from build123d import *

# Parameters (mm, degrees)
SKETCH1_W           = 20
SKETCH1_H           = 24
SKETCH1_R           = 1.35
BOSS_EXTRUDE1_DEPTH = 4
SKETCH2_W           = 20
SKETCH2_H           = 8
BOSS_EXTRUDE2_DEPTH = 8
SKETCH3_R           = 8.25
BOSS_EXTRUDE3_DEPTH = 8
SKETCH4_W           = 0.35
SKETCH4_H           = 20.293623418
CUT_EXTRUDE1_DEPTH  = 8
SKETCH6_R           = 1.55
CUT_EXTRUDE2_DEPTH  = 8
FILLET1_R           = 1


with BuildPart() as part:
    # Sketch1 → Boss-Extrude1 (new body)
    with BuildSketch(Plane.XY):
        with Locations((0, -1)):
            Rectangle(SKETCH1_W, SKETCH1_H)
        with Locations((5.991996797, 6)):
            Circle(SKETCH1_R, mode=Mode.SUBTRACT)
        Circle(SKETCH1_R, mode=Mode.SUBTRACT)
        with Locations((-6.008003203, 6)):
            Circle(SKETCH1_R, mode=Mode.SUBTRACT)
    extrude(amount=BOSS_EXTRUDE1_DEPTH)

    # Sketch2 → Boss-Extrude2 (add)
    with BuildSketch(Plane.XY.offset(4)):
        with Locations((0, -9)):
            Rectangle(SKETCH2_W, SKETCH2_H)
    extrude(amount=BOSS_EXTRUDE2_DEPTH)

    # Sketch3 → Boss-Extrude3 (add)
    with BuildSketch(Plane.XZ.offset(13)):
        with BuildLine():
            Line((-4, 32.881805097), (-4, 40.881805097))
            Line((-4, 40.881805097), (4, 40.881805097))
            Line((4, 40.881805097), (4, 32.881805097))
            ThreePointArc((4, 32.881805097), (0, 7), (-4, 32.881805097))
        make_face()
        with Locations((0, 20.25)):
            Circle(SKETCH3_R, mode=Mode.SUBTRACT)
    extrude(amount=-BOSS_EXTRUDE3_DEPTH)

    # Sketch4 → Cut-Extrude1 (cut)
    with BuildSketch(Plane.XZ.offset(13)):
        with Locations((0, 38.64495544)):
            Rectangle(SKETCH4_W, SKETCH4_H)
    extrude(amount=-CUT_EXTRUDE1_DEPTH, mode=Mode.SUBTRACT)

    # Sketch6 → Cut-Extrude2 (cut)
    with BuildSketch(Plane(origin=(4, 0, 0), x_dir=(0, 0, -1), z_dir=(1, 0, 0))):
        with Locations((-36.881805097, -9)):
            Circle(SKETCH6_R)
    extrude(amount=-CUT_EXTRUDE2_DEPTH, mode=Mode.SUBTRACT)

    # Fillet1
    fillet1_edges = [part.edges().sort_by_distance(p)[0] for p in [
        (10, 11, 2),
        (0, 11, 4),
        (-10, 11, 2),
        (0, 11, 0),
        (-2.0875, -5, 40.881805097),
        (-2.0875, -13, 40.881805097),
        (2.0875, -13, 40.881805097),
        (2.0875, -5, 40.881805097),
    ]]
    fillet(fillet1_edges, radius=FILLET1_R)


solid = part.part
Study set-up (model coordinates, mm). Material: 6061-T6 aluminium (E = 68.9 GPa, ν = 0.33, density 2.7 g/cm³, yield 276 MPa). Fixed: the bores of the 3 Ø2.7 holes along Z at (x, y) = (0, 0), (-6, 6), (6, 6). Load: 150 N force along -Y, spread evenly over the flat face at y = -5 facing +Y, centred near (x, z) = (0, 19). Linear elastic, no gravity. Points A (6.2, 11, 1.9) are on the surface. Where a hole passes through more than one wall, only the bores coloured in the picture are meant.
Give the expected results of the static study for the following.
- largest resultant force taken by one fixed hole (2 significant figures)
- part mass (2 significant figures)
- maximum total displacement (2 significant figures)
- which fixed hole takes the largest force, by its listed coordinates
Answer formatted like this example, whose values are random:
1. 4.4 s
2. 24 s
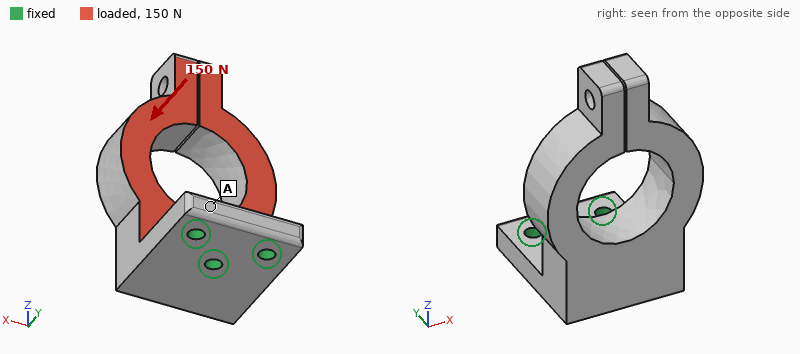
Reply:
1. 210 N
2. 15 g
3. 0.13 mm
4. (0, 0)
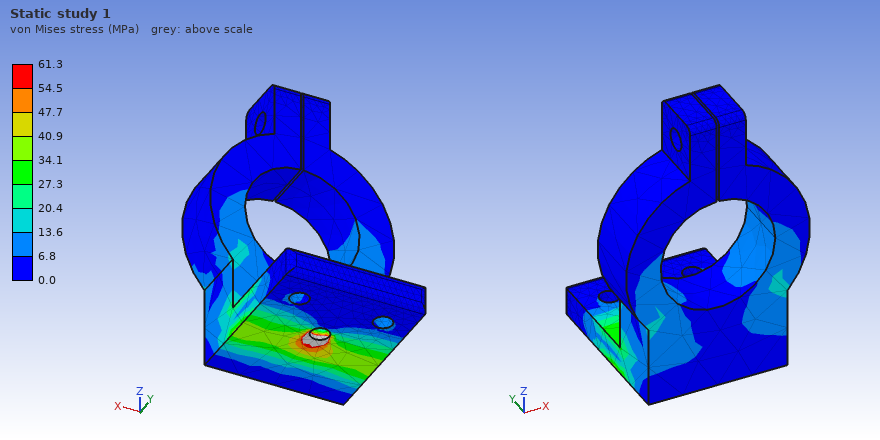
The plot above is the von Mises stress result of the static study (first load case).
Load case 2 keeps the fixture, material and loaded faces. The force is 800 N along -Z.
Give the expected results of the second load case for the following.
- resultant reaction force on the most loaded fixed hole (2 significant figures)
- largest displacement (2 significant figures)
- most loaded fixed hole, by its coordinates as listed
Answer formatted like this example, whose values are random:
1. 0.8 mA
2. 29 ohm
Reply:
1. 850 N
2. 62 µm
3. (0, 0)
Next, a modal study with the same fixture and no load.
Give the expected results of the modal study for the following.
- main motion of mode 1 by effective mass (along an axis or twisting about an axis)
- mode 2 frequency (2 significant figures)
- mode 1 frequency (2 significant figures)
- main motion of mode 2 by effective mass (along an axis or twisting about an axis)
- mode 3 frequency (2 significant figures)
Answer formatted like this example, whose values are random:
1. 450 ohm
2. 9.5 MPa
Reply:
1. along Y
2. 2700 Hz
3. 2100 Hz
4. along X
5. 4100 Hz
